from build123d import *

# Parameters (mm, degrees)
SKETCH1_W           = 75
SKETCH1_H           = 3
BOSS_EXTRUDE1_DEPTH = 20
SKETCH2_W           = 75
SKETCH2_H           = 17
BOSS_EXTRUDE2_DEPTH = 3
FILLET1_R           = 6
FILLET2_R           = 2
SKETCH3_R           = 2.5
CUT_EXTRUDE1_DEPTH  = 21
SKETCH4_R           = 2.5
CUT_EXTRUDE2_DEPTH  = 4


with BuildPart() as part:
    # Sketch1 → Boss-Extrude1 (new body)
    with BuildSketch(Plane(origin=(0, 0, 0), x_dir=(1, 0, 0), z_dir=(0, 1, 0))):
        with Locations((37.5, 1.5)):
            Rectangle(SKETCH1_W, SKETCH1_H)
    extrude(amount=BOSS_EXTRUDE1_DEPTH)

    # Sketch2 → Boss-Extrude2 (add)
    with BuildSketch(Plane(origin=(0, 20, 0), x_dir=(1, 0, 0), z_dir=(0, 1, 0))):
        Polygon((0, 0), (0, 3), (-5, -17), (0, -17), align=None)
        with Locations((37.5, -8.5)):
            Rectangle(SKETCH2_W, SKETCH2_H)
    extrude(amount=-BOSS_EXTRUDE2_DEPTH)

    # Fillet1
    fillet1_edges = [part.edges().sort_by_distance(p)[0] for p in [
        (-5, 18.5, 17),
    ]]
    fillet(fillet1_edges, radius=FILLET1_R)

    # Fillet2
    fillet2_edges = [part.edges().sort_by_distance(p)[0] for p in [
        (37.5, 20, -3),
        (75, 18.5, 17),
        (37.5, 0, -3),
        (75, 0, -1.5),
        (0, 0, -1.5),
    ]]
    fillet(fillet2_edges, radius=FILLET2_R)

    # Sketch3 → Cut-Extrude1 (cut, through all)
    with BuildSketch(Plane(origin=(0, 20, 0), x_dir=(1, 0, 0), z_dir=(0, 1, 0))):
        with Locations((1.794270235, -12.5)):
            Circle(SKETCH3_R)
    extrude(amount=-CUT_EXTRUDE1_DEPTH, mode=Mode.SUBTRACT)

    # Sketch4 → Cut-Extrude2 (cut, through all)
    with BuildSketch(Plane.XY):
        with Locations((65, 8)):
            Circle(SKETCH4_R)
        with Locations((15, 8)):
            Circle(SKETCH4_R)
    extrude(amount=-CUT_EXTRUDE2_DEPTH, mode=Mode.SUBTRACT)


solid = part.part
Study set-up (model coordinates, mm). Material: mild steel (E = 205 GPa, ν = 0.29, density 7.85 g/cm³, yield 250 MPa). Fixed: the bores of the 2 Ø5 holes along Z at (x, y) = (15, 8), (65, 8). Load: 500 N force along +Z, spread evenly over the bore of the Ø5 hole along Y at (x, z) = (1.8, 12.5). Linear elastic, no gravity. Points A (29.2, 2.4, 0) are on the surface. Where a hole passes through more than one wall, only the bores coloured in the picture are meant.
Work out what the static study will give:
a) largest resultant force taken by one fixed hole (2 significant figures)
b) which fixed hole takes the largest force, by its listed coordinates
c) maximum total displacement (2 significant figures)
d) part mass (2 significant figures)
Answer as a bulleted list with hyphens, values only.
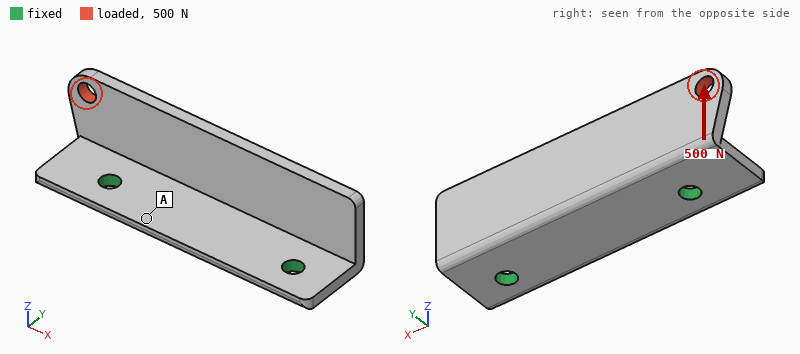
- 620 N
- (15, 8)
- 49 µm
- 64 g
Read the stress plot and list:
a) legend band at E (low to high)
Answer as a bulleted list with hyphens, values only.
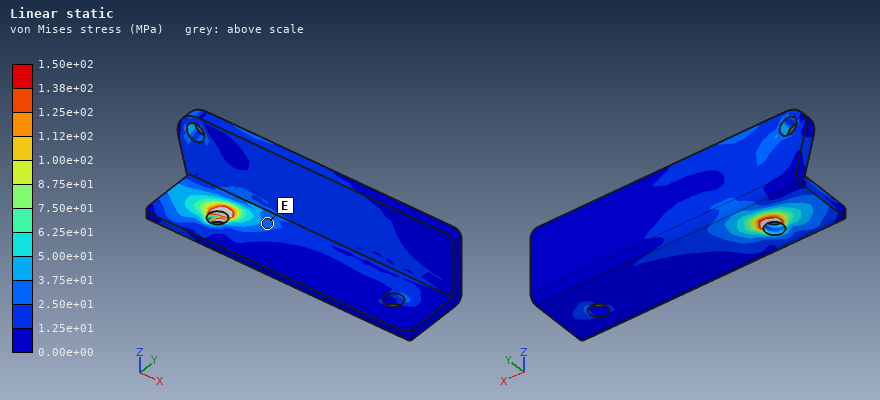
- 2.50e+01 to 3.75e+01 MPa
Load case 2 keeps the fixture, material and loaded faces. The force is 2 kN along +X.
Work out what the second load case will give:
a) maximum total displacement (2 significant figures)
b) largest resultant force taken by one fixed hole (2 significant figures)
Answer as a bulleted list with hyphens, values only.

- 49 µm
- 1.2 kN
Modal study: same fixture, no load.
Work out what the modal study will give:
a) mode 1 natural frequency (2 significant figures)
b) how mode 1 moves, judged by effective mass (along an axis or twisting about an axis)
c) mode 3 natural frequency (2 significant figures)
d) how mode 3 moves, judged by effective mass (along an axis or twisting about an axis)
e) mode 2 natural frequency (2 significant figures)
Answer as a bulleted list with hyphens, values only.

- 3500 Hz
- along Y
- 7900 Hz
- along Z
- 5000 Hz
